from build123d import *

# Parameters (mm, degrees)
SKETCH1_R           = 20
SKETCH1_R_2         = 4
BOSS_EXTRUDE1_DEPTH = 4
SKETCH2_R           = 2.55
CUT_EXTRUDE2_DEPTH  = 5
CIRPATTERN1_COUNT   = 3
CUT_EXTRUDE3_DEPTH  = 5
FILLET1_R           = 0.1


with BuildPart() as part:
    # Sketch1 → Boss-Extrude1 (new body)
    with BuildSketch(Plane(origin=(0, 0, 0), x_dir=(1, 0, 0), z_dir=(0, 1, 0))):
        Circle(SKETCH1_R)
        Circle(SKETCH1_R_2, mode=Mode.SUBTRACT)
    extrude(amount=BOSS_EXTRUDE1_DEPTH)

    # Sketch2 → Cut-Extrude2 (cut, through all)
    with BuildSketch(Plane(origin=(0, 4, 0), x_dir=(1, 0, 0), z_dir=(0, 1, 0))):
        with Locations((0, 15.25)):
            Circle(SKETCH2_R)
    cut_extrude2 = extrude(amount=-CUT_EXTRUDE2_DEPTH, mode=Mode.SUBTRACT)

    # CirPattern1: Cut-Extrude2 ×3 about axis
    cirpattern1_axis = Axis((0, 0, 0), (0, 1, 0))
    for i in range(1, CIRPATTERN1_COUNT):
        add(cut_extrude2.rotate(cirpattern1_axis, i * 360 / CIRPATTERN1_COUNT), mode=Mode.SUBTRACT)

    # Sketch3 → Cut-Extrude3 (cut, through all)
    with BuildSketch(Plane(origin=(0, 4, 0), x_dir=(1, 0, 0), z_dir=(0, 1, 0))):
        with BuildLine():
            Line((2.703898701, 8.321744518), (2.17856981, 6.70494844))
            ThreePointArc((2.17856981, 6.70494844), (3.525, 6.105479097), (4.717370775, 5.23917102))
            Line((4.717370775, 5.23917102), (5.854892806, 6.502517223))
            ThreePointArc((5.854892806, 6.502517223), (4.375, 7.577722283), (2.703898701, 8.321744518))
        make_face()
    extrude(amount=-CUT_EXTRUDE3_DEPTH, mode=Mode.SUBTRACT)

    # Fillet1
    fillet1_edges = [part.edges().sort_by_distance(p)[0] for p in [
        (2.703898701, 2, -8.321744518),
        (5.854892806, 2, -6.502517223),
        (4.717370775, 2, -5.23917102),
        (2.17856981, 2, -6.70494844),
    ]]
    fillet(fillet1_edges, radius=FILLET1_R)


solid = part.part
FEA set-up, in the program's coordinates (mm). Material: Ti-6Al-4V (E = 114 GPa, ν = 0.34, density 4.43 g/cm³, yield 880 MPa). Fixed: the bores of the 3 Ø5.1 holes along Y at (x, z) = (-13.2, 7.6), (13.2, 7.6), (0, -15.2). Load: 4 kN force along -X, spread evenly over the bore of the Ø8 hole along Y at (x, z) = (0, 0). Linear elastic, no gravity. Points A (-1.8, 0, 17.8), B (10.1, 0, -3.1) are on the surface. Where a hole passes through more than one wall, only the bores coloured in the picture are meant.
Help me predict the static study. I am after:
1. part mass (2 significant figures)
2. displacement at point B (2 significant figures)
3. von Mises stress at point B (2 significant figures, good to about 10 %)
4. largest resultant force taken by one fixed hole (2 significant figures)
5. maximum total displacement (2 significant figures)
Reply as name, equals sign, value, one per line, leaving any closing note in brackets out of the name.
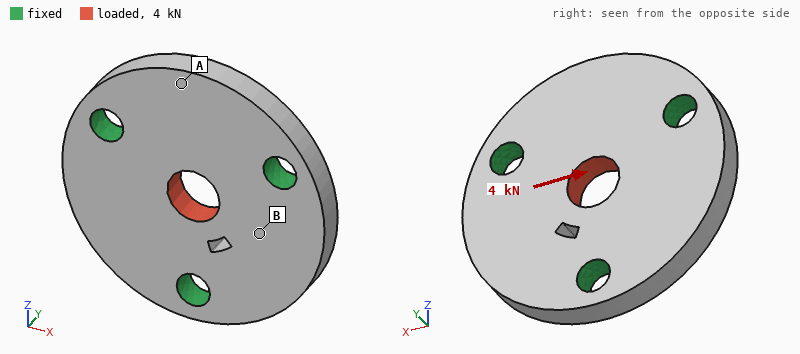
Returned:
part mass = 20 g
displacement at point B = 3.2 µm
von Mises stress at point B = 20 MPa
largest resultant force taken by one fixed hole = 1.4 kN
maximum total displacement = 5.6 µm
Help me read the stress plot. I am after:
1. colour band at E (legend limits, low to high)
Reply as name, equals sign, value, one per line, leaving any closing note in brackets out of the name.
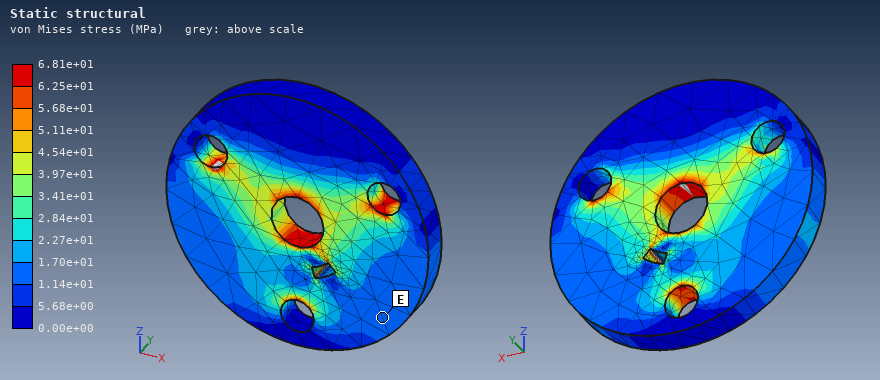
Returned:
colour band at E = 1.14e+01 to 1.70e+01 MPa
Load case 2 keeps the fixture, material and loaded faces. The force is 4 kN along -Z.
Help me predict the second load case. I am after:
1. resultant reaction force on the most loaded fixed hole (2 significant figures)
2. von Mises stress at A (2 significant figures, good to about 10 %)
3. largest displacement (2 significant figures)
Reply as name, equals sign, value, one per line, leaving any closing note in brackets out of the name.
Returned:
resultant reaction force on the most loaded fixed hole = 1.4 kN
von Mises stress at A = 17 MPa
largest displacement = 5.5 µm
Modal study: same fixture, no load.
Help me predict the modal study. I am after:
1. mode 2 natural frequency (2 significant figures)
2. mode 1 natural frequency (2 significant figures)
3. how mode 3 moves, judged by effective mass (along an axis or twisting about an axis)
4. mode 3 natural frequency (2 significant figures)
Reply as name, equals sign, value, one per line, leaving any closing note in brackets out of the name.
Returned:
mode 2 natural frequency = 20 kHz
mode 1 natural frequency = 20 kHz
how mode 3 moves, judged by effective mass = along Y
mode 3 natural frequency = 21 kHz
